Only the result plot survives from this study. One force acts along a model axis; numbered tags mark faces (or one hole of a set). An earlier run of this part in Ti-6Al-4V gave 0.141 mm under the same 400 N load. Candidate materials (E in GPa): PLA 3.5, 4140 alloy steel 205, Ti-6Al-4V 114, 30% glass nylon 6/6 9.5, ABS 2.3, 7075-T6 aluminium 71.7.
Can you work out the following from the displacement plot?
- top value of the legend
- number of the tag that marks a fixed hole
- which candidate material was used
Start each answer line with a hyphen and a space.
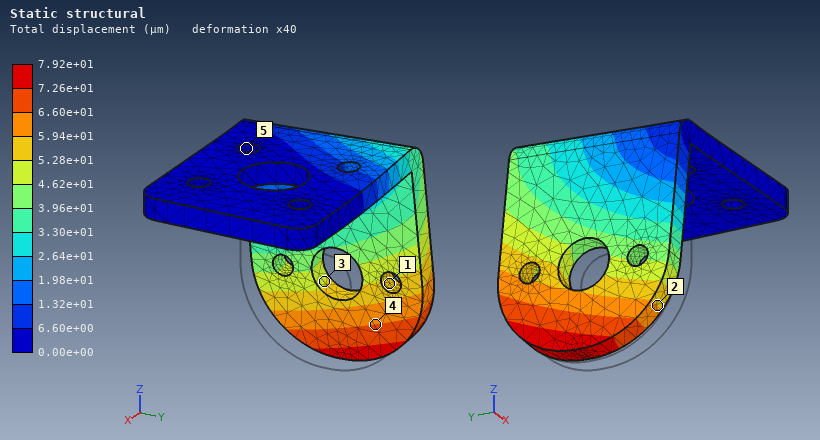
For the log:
- 7.92e+01 µm
- 5
- 4140 alloy steel
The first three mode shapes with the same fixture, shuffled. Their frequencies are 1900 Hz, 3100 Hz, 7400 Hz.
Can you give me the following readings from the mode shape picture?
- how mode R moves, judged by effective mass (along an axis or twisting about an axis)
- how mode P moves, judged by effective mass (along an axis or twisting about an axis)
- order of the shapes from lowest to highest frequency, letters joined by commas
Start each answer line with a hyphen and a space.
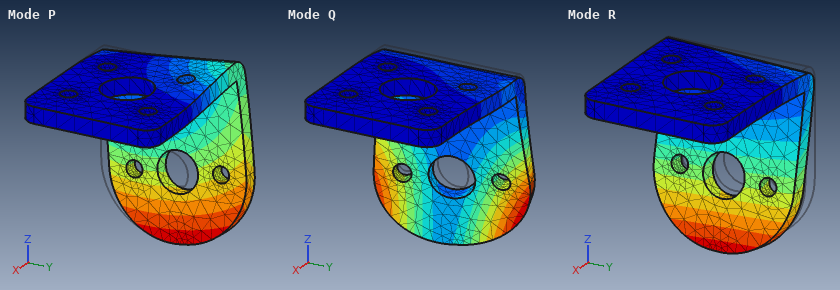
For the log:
- along X
- along Y
- R, P, Q
